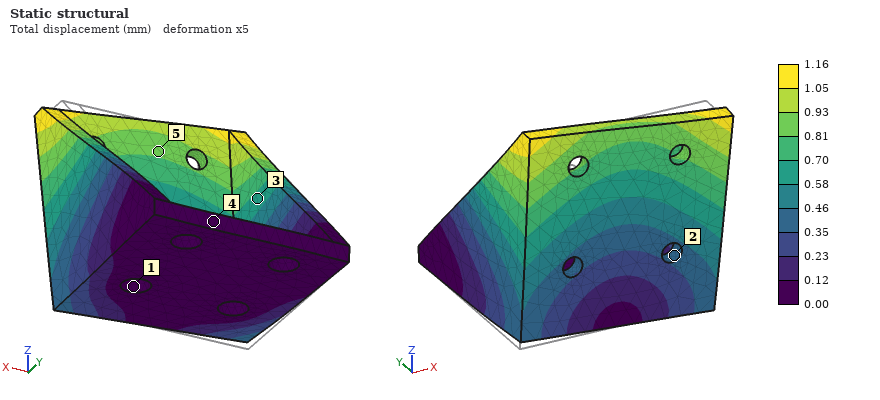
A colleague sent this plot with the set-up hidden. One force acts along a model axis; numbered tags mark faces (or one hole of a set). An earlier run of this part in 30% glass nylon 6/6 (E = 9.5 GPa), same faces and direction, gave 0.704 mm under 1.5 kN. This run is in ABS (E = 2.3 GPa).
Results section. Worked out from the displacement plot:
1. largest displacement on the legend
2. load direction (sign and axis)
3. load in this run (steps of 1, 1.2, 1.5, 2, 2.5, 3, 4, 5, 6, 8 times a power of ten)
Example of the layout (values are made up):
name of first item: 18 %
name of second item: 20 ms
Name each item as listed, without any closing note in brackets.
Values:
largest displacement on the legend: 1.16 mm
load direction: +X
load in this run: 600 N
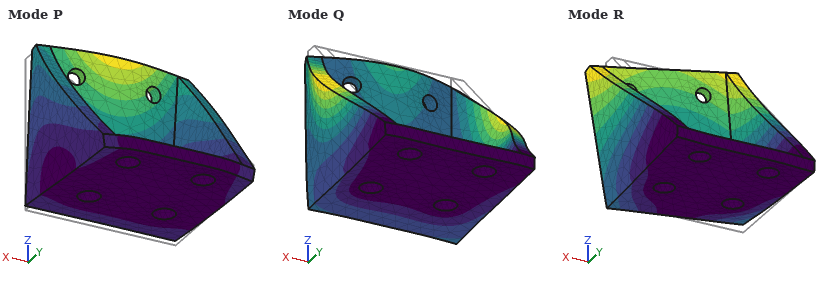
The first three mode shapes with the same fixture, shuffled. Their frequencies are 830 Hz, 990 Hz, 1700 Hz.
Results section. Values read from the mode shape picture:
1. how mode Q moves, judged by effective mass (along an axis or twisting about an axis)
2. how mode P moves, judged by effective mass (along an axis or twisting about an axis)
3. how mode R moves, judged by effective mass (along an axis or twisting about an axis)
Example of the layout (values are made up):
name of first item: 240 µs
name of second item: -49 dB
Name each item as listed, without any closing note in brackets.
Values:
how mode Q moves, judged by effective mass: along Z
how mode P moves, judged by effective mass: along Y
how mode R moves, judged by effective mass: along X
